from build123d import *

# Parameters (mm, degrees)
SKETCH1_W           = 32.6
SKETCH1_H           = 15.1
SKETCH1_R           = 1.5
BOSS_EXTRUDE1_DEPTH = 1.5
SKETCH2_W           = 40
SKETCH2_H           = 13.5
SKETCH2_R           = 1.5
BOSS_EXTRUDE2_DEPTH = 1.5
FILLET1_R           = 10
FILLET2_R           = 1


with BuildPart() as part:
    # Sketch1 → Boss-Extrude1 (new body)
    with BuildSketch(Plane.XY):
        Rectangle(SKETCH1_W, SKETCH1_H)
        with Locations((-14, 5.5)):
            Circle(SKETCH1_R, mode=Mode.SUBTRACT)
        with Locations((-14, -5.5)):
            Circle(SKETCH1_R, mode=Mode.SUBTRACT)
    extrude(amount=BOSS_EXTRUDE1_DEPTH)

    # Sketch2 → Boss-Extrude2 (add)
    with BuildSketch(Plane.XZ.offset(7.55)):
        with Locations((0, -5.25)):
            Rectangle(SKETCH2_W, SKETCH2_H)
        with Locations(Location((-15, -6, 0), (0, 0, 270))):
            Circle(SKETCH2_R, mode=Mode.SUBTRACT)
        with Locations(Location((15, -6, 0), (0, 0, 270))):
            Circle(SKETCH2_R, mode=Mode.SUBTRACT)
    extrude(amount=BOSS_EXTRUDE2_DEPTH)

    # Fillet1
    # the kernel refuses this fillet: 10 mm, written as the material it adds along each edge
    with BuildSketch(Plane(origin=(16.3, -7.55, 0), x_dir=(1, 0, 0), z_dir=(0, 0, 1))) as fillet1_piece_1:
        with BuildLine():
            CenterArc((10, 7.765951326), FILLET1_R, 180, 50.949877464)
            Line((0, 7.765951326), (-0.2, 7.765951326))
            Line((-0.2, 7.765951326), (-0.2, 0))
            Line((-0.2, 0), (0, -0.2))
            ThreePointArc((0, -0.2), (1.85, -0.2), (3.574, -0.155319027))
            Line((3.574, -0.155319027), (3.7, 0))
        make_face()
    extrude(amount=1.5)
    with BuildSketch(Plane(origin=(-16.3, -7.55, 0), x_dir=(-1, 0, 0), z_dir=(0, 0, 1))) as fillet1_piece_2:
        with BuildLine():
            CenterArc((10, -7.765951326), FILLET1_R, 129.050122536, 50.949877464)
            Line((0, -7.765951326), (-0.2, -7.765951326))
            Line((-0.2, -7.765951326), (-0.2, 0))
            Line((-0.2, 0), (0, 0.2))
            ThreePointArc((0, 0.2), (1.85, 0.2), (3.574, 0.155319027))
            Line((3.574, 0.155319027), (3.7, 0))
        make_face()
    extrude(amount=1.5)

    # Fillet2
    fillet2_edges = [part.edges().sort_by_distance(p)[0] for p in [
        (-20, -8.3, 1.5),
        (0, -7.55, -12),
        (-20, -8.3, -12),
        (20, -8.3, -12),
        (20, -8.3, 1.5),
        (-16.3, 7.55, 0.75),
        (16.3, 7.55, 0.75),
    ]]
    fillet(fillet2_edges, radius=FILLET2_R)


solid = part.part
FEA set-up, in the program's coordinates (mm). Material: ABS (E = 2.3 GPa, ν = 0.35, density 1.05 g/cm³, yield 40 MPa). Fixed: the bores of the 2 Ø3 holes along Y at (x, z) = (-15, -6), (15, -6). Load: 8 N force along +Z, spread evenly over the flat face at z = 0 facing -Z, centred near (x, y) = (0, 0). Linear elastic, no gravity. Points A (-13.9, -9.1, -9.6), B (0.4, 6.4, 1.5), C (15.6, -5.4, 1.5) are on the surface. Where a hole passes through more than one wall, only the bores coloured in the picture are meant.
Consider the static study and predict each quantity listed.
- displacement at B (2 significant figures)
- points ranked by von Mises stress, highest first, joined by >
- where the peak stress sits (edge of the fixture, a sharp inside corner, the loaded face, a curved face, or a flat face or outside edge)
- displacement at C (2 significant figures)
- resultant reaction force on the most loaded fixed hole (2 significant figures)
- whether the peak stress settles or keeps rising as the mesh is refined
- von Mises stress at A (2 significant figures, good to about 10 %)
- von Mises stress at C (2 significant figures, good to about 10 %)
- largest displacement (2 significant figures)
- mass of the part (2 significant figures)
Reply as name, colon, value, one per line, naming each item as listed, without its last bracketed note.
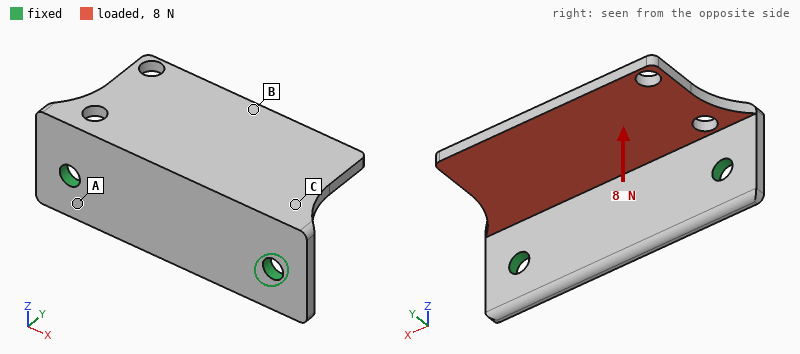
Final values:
displacement at B: 0.42 mm
points ranked by von Mises stress, highest first, joined by >: C > A > B
where the peak stress sits: edge of the fixture
displacement at C: 0.094 mm
resultant reaction force on the most loaded fixed hole: 4.2 N
whether the peak stress settles or keeps rising as the mesh is refined: keeps rising
von Mises stress at A: 2.2 MPa
von Mises stress at C: 3.4 MPa
largest displacement: 0.46 mm
mass of the part: 1.6 g
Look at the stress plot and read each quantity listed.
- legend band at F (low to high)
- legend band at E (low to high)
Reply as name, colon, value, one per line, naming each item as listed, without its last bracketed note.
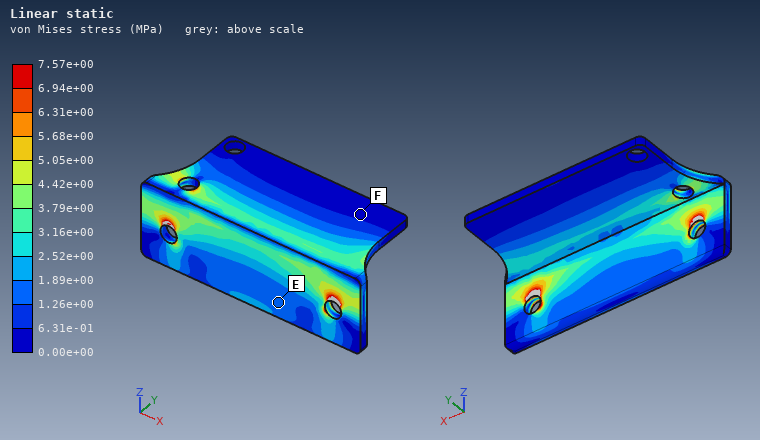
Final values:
legend band at F: 0.00e+00 to 6.31e-01 MPa
legend band at E: 1.26e+00 to 1.89e+00 MPa
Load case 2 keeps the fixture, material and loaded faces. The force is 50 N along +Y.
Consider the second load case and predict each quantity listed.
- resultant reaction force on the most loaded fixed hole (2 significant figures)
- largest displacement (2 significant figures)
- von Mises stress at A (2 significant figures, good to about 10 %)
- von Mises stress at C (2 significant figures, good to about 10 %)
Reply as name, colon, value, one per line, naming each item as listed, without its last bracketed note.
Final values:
resultant reaction force on the most loaded fixed hole: 26 N
largest displacement: 0.52 mm
von Mises stress at A: 3.0 MPa
von Mises stress at C: 2.7 MPa
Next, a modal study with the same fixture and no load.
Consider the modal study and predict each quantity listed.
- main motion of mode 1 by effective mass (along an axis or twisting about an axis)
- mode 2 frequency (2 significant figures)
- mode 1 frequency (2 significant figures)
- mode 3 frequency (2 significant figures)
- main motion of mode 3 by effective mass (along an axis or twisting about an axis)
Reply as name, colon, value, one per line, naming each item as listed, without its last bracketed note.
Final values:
main motion of mode 1 by effective mass: along Z
mode 2 frequency: 1800 Hz
mode 1 frequency: 910 Hz
mode 3 frequency: 2800 Hz
main motion of mode 3 by effective mass: along Y
